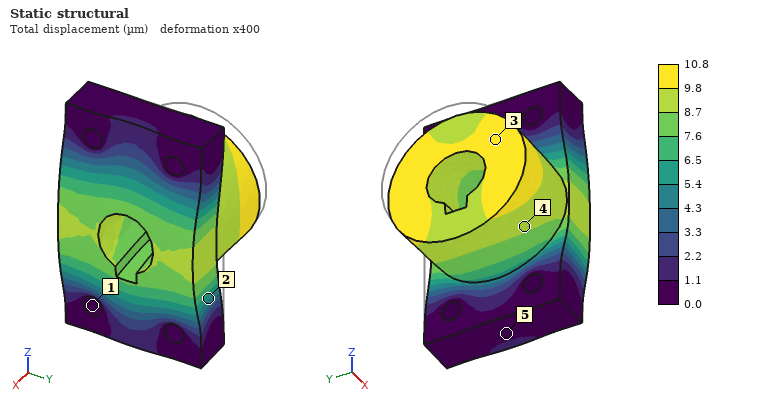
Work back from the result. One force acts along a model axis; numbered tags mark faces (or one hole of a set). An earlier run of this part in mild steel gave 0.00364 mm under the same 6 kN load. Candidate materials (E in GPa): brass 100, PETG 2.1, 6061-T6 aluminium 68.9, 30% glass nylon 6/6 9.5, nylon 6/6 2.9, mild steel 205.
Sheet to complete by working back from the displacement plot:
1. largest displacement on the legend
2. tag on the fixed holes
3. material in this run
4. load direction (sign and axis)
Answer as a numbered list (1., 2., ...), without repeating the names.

1. 10.8 µm
2. 1
3. 6061-T6 aluminium
4. +X
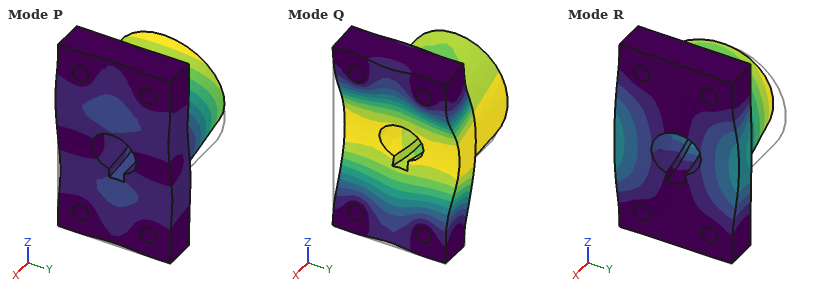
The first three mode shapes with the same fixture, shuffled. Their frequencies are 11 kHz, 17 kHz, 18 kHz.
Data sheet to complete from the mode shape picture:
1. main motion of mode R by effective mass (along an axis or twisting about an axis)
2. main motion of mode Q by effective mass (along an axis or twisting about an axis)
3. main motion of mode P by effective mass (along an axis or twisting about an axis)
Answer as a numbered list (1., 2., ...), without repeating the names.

1. along Y
2. along X
3. along Z
